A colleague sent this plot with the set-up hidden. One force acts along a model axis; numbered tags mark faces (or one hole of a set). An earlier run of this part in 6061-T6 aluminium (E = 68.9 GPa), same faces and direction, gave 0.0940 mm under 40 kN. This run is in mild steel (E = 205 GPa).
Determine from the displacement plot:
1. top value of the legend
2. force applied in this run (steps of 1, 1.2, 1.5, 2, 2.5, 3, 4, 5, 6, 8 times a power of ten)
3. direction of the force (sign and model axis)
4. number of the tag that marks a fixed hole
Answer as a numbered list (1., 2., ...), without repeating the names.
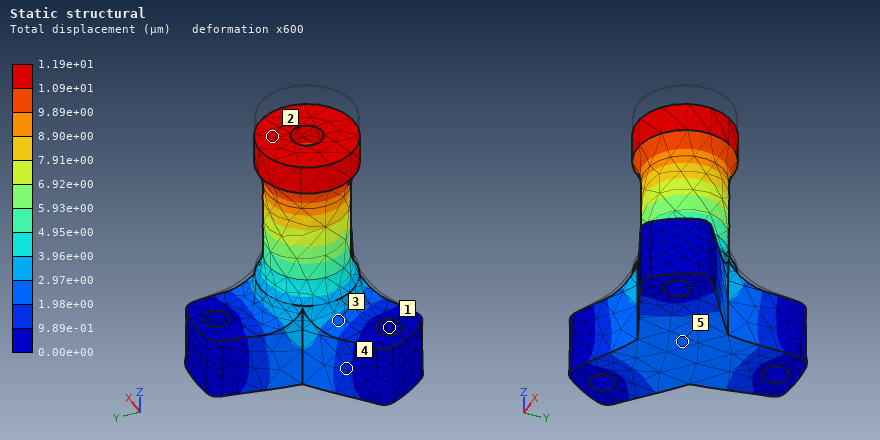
1. 1.19e+01 µm
2. 15 kN
3. -Z
4. 1
